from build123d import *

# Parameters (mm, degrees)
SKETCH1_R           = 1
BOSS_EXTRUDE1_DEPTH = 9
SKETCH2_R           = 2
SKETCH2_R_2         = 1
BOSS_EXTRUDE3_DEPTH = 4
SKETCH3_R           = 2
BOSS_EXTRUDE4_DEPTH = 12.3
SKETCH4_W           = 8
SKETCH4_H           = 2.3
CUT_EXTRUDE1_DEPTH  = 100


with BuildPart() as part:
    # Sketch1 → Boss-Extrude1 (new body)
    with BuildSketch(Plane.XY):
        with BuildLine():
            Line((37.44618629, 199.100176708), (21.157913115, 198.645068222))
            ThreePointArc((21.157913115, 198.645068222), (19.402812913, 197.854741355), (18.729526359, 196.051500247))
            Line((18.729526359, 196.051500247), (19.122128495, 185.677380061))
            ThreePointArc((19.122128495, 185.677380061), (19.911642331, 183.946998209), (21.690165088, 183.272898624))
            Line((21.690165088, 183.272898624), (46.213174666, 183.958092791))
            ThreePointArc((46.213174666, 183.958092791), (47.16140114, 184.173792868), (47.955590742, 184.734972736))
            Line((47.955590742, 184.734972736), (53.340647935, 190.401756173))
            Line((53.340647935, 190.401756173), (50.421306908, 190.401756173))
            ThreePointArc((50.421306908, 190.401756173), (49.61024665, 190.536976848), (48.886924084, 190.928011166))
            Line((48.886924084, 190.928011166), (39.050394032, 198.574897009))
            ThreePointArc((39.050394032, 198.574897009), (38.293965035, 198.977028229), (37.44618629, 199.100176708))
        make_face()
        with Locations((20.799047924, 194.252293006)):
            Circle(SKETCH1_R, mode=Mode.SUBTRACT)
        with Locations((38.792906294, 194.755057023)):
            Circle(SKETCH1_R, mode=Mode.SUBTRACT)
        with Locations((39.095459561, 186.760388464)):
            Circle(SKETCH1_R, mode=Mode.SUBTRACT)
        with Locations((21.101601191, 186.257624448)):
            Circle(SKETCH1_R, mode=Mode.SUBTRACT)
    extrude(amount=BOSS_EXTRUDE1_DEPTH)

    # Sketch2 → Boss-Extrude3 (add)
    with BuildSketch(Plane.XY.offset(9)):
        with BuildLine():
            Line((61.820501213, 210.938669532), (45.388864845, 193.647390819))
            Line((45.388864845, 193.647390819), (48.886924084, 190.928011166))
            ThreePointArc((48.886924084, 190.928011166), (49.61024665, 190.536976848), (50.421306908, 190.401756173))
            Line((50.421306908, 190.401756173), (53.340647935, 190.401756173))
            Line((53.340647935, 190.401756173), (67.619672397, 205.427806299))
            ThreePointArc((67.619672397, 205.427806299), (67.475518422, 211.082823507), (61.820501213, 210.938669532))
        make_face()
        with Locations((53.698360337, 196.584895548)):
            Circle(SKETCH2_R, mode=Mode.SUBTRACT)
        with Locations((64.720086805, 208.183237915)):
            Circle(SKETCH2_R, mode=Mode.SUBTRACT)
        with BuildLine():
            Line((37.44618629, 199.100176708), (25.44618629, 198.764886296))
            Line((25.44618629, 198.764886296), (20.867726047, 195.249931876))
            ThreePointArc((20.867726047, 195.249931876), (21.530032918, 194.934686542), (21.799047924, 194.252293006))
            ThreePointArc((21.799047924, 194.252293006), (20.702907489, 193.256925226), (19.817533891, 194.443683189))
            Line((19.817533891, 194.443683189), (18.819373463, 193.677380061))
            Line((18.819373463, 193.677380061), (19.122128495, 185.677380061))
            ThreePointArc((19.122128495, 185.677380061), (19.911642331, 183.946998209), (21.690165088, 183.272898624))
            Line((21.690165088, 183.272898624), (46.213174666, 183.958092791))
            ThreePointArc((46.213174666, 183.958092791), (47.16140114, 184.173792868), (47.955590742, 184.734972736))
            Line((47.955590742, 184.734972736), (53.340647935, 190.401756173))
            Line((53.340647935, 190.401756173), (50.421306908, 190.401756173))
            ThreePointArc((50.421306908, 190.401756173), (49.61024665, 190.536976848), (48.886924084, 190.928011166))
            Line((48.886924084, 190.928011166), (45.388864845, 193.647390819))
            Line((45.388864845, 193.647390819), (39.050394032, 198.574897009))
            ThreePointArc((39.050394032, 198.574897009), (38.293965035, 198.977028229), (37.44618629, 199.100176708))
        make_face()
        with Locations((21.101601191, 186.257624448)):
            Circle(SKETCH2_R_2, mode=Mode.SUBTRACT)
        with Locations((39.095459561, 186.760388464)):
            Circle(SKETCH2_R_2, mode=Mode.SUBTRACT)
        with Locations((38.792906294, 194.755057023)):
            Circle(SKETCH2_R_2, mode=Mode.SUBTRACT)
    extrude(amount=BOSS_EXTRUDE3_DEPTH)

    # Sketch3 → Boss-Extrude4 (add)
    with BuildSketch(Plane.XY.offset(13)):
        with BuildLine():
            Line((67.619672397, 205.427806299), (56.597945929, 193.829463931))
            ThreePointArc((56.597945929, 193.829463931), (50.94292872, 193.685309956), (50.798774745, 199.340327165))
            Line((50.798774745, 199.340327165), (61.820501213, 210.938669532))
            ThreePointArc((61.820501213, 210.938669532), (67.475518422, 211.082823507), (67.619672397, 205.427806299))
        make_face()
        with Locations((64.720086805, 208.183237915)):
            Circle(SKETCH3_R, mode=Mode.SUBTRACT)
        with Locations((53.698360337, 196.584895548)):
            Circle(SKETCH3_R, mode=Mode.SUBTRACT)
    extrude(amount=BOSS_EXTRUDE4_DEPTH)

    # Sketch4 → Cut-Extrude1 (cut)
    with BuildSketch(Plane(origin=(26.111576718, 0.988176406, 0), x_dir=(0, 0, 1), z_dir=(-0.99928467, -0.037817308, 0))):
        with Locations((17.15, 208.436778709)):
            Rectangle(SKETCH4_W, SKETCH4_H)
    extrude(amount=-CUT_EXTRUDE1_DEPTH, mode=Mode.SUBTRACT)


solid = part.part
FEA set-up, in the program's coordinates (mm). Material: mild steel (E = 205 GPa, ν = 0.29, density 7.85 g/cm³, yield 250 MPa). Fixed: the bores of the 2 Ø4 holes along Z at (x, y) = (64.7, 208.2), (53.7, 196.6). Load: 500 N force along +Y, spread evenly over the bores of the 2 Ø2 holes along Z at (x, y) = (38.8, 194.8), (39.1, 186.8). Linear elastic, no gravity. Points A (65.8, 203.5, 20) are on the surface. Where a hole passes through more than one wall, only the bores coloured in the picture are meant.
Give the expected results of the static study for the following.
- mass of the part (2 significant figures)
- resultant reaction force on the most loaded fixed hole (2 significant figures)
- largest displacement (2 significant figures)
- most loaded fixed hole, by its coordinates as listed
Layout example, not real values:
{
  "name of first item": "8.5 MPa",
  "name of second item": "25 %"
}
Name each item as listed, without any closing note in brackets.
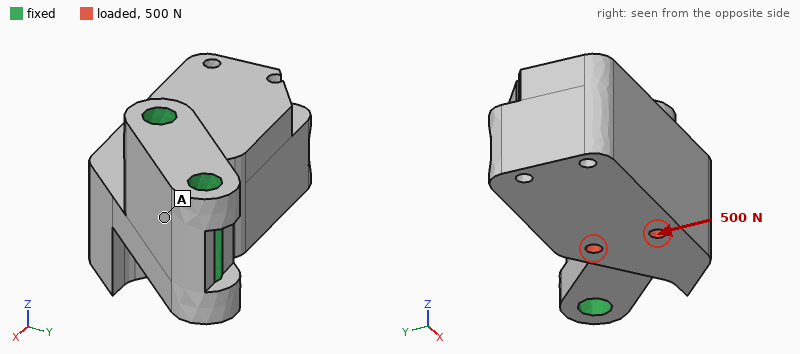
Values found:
{
  "mass of the part": "61 g",
  "resultant reaction force on the most loaded fixed hole": "550 N",
  "largest displacement": "74 µm",
  "most loaded fixed hole, by its coordinates as listed": "(53.7, 196.6)"
}
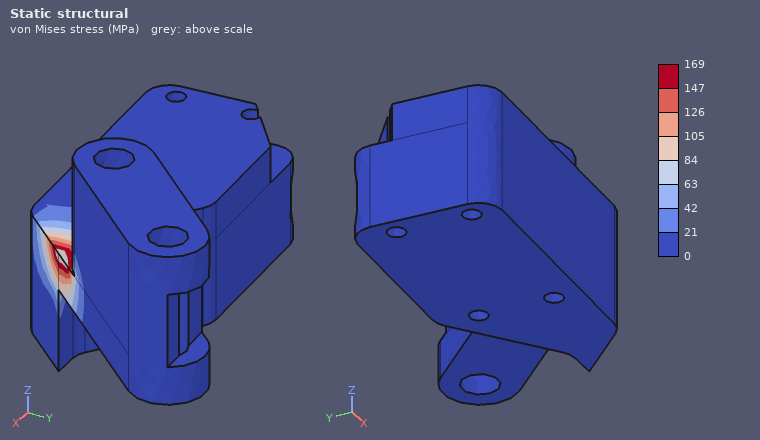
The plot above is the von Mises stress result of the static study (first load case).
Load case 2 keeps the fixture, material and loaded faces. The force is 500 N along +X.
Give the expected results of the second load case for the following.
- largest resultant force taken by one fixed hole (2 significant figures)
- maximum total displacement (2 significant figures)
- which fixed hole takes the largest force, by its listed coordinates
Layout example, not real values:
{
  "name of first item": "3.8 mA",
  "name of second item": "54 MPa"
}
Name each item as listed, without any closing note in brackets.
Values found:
{
  "largest resultant force taken by one fixed hole": "520 N",
  "maximum total displacement": "46 µm",
  "which fixed hole takes the largest force, by its listed coordinates": "(53.7, 196.6)"
}
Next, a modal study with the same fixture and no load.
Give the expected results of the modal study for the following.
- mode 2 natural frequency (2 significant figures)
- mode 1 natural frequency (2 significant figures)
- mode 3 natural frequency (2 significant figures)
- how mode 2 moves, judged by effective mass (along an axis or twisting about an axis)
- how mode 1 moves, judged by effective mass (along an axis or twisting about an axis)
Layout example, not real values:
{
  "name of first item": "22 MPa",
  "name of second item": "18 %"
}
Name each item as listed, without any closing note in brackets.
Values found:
{
  "mode 2 natural frequency": "2200 Hz",
  "mode 1 natural frequency": "1600 Hz",
  "mode 3 natural frequency": "5000 Hz",
  "how mode 2 moves, judged by effective mass": "along Y",
  "how mode 1 moves, judged by effective mass": "along Z"
}
